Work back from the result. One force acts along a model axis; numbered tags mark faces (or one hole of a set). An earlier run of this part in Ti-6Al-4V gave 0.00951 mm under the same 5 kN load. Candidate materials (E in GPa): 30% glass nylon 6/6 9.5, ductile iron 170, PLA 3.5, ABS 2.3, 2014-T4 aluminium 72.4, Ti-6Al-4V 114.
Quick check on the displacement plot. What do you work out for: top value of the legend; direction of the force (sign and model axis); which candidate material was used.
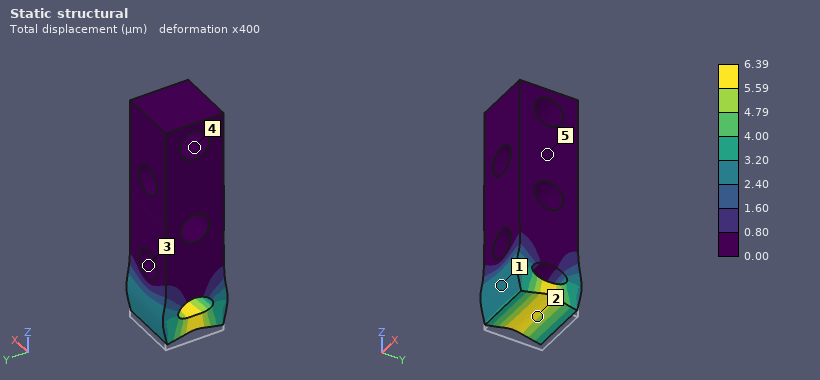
6.39 µm
+Z
ductile iron
